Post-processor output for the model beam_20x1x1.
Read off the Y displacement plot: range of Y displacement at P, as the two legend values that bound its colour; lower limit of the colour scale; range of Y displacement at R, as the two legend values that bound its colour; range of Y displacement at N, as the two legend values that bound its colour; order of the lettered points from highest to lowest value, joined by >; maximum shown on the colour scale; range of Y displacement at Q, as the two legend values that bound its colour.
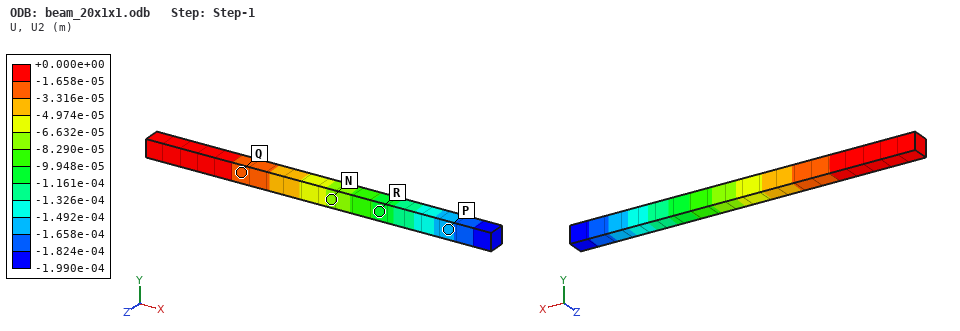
-1.658e-04 to -1.492e-04 m
-1.990e-04 m
-1.161e-04 to -9.948e-05 m
-8.290e-05 to -6.632e-05 m
Q > N > R > P
+0.000e+00 m
-3.316e-05 to -1.658e-05 m
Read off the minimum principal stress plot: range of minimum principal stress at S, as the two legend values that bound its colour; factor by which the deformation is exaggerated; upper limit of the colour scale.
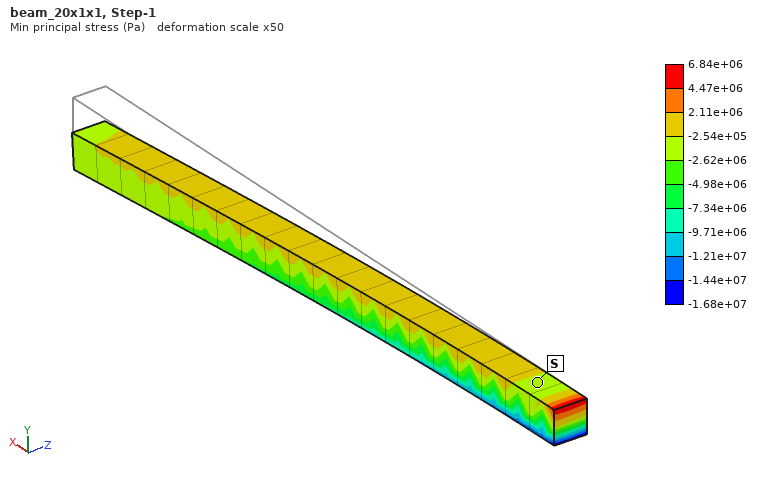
-2.62e+06 to -2.54e+05 Pa
50
6.84e+06 Pa
